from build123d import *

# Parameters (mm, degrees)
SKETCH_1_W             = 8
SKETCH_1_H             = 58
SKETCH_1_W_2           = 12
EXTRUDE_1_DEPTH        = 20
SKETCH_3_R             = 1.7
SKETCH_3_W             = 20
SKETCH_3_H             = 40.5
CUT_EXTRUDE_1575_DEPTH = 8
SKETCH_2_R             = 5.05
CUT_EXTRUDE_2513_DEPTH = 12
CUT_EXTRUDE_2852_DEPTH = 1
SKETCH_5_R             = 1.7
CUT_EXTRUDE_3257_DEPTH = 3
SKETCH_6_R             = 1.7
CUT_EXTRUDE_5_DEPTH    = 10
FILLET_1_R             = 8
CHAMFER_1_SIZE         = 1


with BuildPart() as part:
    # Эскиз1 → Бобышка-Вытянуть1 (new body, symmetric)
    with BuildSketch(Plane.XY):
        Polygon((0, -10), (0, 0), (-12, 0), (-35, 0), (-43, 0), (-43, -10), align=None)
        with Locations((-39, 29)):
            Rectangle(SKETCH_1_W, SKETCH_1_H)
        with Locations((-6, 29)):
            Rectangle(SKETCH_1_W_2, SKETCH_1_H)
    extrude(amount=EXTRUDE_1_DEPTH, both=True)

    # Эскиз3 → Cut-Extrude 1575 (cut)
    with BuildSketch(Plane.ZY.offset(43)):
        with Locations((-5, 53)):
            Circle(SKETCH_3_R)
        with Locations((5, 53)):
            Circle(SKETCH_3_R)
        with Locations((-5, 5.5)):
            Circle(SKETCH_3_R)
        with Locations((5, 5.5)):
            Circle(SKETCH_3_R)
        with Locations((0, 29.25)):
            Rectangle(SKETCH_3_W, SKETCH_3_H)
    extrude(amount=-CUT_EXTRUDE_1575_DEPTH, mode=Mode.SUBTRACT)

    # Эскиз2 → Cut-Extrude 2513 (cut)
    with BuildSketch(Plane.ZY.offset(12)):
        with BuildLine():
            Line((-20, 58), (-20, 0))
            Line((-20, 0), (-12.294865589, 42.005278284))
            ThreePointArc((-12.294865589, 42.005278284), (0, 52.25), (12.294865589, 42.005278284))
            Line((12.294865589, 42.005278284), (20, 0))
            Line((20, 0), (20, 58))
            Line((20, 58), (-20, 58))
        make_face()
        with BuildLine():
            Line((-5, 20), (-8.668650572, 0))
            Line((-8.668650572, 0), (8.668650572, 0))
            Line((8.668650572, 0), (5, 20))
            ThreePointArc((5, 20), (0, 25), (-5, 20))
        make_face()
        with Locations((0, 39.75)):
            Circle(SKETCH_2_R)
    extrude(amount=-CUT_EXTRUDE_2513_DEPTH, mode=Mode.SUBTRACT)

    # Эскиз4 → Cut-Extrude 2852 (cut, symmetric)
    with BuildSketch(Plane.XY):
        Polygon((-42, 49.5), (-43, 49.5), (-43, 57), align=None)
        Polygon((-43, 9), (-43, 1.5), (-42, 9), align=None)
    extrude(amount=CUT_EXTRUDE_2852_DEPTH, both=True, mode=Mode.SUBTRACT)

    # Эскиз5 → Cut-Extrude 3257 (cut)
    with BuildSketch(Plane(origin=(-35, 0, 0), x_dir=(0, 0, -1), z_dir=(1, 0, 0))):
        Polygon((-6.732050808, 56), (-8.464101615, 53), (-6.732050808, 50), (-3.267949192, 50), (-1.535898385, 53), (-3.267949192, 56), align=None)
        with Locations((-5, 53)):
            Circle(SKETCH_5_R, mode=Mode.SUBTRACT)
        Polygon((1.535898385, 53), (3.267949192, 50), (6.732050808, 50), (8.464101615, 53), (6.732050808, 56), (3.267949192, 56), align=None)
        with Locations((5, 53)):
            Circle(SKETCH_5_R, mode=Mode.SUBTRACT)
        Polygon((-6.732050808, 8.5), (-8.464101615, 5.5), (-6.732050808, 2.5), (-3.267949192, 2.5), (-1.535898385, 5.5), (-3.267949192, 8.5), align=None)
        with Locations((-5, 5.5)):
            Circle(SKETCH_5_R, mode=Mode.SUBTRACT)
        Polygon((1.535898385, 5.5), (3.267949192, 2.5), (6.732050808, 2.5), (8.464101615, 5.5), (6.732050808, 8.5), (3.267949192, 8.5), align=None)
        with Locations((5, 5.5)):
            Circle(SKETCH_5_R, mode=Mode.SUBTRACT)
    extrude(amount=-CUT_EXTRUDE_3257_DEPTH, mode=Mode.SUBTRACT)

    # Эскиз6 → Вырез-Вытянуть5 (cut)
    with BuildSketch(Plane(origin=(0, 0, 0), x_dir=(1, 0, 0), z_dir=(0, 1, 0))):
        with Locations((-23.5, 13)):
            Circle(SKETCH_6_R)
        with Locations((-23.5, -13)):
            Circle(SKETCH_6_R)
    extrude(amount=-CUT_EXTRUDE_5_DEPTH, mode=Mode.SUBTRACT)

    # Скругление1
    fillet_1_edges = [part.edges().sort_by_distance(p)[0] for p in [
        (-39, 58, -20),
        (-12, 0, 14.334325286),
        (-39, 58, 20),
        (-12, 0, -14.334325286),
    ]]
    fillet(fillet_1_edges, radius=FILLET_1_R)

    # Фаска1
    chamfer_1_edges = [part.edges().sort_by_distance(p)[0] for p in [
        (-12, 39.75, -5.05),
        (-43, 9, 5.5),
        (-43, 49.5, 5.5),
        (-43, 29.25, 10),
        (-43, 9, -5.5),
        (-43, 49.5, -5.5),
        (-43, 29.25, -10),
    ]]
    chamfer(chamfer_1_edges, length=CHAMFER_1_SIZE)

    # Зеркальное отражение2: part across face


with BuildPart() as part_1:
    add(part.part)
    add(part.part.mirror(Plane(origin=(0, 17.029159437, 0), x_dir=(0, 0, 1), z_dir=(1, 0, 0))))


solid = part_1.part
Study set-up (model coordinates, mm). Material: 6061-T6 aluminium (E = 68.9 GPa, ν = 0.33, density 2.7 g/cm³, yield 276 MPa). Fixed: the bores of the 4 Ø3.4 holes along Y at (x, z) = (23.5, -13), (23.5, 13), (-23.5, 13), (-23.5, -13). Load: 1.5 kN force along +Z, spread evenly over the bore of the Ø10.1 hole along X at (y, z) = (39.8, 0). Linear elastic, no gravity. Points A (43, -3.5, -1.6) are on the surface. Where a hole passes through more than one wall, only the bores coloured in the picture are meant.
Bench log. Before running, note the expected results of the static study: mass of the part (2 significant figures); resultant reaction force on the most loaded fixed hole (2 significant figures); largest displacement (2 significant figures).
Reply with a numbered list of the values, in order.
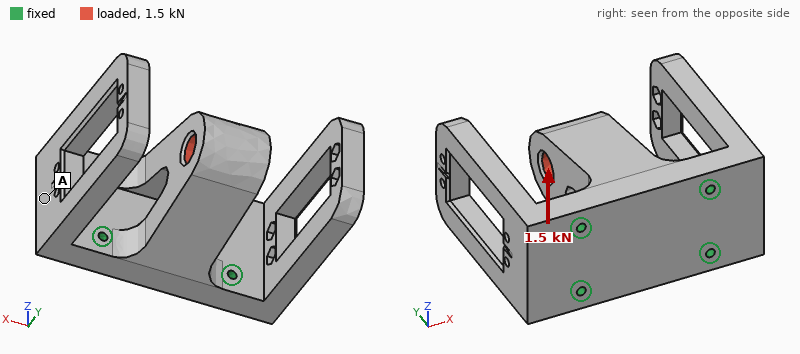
1. 230 g
2. 1.3 kN
3. 46 µm
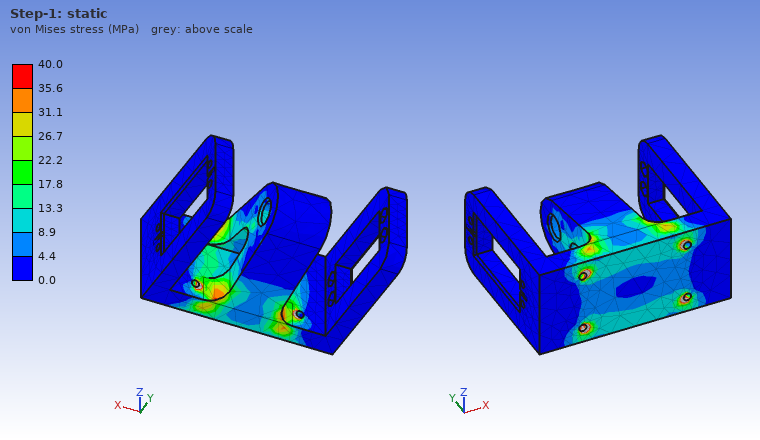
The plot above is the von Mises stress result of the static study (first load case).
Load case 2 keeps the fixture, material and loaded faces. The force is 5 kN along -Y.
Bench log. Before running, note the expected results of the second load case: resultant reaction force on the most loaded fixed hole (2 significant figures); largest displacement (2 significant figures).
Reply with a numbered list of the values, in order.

1. 1.3 kN
2. 15 µm
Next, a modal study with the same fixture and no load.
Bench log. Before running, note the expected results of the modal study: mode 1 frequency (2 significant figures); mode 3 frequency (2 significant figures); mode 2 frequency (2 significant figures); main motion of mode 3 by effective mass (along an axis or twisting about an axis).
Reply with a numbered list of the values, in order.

1. 1400 Hz
2. 2700 Hz
3. 1400 Hz
4. along Z
